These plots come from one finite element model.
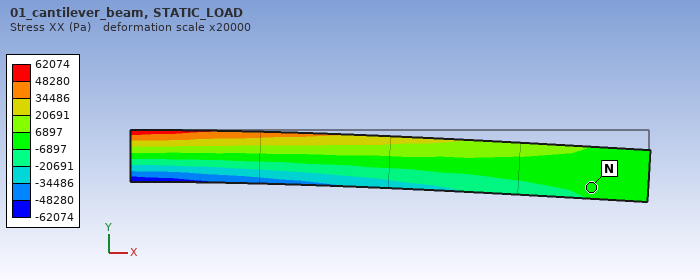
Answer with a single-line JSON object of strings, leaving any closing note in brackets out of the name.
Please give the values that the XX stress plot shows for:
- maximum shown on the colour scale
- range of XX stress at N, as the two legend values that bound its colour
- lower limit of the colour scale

{"maximum shown on the colour scale": "62074 Pa", "range of XX stress at N, as the two legend values that bound its colour": "-6897 to 6897 Pa", "lower limit of the colour scale": "-62074 Pa"}
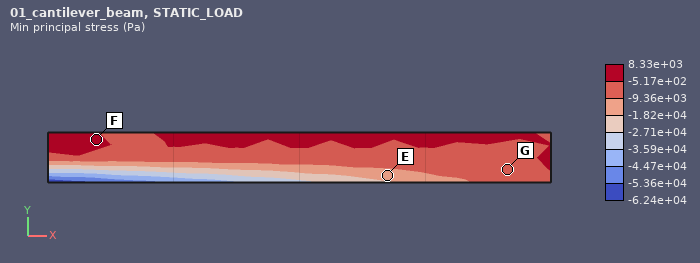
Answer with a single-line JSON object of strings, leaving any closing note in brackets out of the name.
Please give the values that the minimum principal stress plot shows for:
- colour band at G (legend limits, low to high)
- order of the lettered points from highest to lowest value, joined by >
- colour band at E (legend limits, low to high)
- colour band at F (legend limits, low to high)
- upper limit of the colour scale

{"colour band at G": "-9.36e+03 to -5.17e+02 Pa", "order of the lettered points from highest to lowest value, joined by >": "F > G > E", "colour band at E": "-1.82e+04 to -9.36e+03 Pa", "colour band at F": "-5.17e+02 to 8.33e+03 Pa", "upper limit of the colour scale": "8.33e+03 Pa"}
